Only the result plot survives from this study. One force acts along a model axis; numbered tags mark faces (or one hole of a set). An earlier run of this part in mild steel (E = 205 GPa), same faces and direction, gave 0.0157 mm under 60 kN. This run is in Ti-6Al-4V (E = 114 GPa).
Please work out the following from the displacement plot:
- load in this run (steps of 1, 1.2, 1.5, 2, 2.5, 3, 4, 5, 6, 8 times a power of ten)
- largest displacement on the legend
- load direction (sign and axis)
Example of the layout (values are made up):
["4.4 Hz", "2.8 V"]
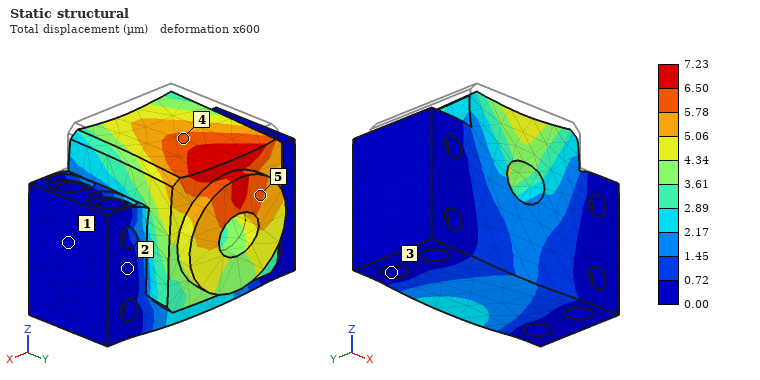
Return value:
["15 kN", "7.23 µm", "-Z"]
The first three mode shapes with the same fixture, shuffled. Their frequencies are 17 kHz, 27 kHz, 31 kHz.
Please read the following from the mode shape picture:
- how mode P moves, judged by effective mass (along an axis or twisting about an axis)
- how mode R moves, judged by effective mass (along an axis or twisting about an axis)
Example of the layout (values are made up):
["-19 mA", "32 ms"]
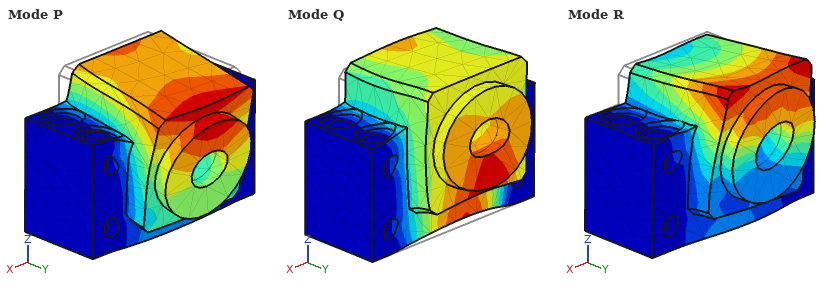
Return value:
["along Y", "along X"]
